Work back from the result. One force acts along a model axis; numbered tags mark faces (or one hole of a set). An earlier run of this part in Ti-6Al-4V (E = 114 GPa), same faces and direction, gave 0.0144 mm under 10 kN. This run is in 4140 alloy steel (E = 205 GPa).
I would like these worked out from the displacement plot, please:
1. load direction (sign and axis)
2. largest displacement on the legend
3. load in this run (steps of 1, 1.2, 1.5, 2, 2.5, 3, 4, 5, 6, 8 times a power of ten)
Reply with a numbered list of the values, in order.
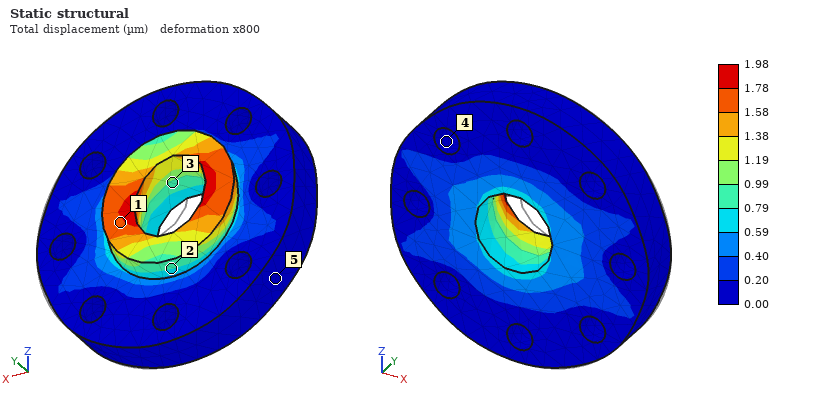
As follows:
1. -X
2. 1.98 µm
3. 2.5 kN
